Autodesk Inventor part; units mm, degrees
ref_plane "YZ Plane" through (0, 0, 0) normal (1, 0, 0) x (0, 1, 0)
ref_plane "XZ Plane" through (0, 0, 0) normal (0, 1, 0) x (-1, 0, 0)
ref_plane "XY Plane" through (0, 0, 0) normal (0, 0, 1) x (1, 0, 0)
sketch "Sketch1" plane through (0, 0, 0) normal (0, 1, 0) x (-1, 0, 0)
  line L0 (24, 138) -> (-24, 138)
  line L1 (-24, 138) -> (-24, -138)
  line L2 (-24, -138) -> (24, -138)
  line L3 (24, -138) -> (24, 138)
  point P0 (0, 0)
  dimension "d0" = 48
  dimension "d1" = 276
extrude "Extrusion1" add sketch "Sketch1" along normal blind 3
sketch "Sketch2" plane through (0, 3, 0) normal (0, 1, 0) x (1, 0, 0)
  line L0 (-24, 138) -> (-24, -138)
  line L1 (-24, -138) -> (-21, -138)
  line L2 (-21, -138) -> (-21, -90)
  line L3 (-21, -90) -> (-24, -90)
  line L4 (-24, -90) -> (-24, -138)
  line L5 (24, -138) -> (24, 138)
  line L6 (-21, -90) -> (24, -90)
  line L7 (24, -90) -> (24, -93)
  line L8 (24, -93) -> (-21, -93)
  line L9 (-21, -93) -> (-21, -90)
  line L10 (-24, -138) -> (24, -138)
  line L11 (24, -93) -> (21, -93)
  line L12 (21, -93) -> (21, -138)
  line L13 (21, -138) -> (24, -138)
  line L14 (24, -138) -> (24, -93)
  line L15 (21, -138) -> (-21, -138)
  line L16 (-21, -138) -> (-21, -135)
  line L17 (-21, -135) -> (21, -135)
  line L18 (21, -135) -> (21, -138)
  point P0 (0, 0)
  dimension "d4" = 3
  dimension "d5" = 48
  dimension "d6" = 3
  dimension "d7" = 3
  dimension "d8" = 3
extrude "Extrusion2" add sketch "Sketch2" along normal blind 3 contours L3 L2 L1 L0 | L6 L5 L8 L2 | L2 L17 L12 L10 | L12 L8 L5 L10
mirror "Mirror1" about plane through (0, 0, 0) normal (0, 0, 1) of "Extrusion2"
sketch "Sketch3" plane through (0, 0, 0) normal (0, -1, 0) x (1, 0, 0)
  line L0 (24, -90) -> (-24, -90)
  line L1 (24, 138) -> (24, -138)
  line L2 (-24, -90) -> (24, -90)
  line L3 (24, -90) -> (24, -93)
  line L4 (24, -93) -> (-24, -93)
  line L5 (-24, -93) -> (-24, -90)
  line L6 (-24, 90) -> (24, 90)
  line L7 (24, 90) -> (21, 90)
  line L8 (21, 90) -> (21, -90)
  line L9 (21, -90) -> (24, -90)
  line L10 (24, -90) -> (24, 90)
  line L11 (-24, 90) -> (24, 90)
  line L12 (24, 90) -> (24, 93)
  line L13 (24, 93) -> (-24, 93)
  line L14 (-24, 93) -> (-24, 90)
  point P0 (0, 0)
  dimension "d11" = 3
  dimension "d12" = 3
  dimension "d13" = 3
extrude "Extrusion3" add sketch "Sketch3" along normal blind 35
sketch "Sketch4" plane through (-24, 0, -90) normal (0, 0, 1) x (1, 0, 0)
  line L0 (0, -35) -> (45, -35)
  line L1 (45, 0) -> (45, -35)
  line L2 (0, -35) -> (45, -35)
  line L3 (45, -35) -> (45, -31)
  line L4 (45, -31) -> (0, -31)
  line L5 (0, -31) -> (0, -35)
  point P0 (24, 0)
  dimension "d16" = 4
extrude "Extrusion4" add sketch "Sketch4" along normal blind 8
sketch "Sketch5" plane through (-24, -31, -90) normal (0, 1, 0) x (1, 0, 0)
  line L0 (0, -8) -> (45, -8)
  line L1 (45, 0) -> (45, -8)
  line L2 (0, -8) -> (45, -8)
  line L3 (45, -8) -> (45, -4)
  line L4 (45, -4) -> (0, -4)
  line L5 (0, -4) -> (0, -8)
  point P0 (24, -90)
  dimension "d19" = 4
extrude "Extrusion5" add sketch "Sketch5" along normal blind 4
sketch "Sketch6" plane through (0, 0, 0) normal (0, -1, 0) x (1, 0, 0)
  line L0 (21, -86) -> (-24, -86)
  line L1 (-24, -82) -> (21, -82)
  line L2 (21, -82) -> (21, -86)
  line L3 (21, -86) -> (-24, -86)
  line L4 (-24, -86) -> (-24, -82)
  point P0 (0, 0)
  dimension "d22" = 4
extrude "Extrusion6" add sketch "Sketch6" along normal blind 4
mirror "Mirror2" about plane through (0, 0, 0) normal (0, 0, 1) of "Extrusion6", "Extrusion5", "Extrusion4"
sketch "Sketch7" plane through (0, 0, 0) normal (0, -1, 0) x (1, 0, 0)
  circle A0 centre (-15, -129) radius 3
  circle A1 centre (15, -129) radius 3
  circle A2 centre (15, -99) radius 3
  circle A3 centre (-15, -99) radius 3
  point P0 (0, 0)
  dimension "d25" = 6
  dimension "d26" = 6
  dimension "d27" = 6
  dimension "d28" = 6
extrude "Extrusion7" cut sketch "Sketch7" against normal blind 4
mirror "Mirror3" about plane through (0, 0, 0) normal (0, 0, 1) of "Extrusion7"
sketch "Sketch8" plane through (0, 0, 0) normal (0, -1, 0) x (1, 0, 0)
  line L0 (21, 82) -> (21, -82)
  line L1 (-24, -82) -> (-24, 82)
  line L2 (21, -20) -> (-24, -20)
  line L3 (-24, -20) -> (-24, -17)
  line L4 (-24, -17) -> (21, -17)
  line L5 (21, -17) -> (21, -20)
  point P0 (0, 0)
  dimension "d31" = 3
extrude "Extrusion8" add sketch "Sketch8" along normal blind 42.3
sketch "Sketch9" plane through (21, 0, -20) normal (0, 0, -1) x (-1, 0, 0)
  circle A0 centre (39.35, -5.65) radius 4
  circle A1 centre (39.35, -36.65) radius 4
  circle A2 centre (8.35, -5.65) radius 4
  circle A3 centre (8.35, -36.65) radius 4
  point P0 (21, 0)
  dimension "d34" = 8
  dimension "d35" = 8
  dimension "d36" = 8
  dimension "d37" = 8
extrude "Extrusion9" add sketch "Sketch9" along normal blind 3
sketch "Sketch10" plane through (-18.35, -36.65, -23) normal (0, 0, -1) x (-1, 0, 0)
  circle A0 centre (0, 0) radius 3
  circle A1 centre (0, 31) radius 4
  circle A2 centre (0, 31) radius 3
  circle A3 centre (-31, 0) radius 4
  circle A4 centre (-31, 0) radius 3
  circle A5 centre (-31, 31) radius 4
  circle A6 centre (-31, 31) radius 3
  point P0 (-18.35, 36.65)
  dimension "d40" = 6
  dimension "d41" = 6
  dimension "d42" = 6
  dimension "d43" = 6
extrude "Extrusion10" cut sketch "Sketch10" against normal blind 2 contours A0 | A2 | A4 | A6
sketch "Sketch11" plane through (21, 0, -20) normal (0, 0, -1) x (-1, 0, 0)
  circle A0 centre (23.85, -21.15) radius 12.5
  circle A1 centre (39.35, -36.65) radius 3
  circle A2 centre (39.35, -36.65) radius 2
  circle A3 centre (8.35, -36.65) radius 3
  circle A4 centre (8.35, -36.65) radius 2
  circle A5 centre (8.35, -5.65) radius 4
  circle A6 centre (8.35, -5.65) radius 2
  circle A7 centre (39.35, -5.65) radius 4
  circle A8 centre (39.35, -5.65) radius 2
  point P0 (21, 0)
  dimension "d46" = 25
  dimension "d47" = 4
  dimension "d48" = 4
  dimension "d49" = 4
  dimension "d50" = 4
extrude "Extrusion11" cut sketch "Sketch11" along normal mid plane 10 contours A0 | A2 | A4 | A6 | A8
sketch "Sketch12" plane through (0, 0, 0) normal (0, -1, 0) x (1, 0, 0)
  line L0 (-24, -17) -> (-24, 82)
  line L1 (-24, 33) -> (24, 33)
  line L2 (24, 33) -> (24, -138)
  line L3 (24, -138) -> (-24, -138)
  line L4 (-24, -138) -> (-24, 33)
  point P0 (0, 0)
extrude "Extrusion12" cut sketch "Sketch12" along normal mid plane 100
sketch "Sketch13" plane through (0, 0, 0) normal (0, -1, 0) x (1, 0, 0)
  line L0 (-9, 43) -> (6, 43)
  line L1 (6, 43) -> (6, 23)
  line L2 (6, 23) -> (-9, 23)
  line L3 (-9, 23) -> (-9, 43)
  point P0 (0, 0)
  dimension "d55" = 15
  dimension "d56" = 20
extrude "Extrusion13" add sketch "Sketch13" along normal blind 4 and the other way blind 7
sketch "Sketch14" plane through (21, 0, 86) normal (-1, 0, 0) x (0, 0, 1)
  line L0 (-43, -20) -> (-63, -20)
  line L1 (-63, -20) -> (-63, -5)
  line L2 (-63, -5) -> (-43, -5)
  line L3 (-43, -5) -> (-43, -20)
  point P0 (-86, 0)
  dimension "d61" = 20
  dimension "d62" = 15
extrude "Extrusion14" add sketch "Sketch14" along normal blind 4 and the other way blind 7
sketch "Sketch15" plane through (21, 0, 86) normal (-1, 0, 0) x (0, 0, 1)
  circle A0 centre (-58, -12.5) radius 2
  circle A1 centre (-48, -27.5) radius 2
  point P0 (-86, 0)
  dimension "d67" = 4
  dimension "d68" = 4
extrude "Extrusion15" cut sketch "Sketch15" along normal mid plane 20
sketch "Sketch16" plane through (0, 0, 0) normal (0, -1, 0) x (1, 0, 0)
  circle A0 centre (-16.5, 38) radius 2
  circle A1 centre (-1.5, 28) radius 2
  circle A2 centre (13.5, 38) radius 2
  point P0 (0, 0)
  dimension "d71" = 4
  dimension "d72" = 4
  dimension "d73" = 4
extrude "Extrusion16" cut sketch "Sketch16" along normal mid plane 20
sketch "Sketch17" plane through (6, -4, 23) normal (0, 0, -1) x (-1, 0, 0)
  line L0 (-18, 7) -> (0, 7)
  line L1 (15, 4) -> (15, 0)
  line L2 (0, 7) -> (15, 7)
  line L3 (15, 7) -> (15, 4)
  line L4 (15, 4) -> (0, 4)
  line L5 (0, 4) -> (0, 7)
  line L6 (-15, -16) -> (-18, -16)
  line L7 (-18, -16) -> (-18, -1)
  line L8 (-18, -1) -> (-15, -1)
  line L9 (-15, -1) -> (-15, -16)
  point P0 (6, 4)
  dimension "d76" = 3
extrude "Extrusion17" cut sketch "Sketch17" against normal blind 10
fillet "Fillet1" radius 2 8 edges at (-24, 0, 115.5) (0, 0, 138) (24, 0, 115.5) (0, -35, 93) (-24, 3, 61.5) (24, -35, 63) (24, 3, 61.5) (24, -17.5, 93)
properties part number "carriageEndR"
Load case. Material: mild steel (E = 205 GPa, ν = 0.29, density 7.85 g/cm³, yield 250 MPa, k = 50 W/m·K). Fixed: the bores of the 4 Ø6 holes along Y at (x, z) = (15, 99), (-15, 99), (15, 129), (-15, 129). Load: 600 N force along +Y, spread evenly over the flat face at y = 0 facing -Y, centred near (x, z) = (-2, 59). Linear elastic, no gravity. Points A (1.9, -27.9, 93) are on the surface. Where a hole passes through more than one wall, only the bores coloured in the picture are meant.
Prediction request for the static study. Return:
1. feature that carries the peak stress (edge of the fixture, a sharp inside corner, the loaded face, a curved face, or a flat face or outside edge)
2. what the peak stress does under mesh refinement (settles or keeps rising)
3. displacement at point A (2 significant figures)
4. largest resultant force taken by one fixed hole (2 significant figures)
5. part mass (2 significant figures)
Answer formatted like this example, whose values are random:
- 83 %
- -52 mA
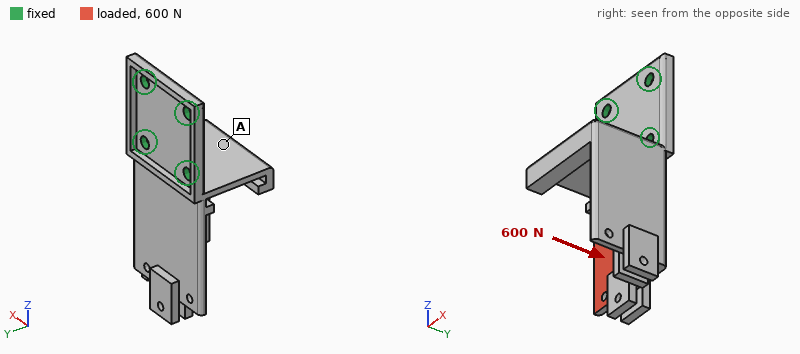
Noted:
- edge of the fixture
- keeps rising
- 0.15 mm
- 640 N
- 270 g
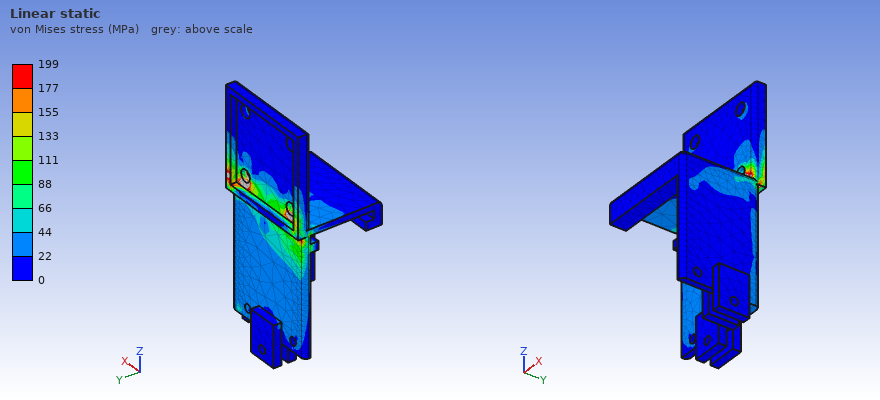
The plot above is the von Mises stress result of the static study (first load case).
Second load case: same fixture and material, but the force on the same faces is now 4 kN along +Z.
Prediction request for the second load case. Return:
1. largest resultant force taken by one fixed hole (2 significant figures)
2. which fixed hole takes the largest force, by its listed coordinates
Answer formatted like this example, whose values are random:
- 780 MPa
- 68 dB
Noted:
- 2.0 kN
- (-15, 99)
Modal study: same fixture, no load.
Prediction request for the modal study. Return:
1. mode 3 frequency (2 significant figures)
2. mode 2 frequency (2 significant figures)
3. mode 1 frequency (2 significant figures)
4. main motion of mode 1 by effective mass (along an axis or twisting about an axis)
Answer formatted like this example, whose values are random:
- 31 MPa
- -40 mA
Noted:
- 2000 Hz
- 1300 Hz
- 490 Hz
- along Y
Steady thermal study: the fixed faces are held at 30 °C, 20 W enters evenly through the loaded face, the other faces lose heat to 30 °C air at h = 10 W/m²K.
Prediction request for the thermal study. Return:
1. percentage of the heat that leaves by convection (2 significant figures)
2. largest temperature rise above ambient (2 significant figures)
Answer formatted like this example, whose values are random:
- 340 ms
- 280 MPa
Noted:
- 28 %
- 70 K
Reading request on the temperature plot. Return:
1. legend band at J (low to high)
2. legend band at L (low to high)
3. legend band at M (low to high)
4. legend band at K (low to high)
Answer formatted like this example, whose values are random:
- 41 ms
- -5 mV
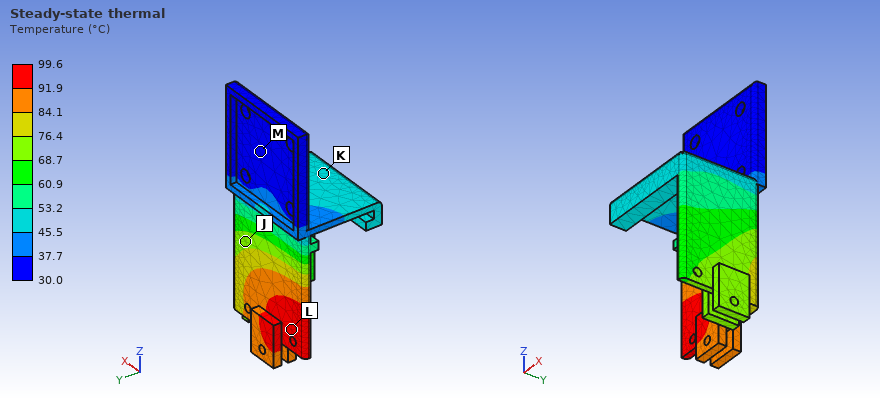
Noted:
- 68.7 to 76.4 °C
- 91.9 to 99.6 °C
- 30.0 to 37.7 °C
- 45.5 to 53.2 °C
